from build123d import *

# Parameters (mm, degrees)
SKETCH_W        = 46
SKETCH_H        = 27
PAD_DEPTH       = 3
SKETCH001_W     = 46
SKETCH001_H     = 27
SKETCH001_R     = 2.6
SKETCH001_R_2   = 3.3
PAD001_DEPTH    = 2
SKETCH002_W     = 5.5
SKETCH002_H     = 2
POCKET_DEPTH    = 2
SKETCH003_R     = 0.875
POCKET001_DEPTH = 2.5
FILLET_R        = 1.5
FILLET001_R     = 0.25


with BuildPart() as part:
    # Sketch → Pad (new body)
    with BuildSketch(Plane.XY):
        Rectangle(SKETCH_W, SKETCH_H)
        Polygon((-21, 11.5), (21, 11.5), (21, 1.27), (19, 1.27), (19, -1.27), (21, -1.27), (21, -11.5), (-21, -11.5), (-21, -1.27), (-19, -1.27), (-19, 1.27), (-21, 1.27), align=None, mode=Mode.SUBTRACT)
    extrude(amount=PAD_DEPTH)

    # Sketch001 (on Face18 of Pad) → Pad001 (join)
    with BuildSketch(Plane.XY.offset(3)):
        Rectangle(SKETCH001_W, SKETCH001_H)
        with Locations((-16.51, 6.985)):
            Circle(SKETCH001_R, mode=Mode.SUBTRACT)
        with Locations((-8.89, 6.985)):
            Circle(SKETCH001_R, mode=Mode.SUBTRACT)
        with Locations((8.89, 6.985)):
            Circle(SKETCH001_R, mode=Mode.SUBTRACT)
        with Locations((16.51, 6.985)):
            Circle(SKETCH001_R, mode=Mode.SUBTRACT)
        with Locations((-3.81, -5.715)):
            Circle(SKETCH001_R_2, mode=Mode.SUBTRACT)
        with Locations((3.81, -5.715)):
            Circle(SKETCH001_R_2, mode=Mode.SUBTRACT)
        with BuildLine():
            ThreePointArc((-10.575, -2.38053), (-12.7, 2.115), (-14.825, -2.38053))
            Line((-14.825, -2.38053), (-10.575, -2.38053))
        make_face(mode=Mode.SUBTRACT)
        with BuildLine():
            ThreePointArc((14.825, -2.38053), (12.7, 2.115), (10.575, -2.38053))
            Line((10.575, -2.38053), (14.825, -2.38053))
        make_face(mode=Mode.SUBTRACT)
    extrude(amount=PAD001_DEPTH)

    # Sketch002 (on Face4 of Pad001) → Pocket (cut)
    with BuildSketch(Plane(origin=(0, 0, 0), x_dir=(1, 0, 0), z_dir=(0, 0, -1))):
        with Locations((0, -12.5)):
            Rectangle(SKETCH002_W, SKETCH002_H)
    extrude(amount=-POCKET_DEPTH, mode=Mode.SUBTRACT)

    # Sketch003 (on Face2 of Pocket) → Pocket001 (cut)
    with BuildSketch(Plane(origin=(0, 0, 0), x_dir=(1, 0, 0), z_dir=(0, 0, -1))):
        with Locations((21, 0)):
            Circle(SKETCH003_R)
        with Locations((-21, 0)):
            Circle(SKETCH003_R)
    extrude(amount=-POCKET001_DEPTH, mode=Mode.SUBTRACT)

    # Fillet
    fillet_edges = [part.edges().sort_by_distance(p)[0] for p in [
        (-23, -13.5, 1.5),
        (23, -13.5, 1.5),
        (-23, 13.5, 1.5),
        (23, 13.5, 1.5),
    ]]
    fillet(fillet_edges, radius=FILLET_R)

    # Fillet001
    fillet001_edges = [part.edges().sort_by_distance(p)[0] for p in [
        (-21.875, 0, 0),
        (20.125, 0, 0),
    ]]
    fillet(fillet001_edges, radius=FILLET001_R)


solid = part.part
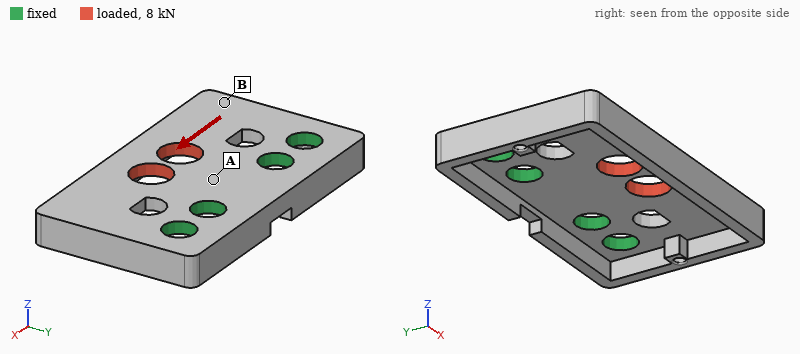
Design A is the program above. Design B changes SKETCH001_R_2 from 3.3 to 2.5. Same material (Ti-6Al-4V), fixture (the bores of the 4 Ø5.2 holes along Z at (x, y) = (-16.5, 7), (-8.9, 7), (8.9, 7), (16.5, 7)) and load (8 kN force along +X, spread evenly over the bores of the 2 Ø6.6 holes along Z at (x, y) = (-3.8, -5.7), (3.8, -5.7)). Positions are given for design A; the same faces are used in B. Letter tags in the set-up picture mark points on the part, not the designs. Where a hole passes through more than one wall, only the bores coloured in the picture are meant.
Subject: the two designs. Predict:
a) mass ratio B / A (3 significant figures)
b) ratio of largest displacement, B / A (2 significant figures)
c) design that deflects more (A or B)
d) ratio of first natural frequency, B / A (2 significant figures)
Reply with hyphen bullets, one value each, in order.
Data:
- 1.02
- 0.70
- A
- 1.0
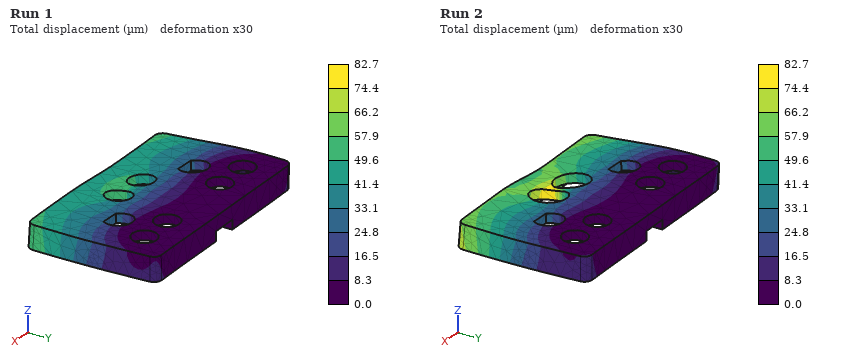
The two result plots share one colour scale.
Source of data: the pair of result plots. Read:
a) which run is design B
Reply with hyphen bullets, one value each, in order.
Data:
- Run 1
